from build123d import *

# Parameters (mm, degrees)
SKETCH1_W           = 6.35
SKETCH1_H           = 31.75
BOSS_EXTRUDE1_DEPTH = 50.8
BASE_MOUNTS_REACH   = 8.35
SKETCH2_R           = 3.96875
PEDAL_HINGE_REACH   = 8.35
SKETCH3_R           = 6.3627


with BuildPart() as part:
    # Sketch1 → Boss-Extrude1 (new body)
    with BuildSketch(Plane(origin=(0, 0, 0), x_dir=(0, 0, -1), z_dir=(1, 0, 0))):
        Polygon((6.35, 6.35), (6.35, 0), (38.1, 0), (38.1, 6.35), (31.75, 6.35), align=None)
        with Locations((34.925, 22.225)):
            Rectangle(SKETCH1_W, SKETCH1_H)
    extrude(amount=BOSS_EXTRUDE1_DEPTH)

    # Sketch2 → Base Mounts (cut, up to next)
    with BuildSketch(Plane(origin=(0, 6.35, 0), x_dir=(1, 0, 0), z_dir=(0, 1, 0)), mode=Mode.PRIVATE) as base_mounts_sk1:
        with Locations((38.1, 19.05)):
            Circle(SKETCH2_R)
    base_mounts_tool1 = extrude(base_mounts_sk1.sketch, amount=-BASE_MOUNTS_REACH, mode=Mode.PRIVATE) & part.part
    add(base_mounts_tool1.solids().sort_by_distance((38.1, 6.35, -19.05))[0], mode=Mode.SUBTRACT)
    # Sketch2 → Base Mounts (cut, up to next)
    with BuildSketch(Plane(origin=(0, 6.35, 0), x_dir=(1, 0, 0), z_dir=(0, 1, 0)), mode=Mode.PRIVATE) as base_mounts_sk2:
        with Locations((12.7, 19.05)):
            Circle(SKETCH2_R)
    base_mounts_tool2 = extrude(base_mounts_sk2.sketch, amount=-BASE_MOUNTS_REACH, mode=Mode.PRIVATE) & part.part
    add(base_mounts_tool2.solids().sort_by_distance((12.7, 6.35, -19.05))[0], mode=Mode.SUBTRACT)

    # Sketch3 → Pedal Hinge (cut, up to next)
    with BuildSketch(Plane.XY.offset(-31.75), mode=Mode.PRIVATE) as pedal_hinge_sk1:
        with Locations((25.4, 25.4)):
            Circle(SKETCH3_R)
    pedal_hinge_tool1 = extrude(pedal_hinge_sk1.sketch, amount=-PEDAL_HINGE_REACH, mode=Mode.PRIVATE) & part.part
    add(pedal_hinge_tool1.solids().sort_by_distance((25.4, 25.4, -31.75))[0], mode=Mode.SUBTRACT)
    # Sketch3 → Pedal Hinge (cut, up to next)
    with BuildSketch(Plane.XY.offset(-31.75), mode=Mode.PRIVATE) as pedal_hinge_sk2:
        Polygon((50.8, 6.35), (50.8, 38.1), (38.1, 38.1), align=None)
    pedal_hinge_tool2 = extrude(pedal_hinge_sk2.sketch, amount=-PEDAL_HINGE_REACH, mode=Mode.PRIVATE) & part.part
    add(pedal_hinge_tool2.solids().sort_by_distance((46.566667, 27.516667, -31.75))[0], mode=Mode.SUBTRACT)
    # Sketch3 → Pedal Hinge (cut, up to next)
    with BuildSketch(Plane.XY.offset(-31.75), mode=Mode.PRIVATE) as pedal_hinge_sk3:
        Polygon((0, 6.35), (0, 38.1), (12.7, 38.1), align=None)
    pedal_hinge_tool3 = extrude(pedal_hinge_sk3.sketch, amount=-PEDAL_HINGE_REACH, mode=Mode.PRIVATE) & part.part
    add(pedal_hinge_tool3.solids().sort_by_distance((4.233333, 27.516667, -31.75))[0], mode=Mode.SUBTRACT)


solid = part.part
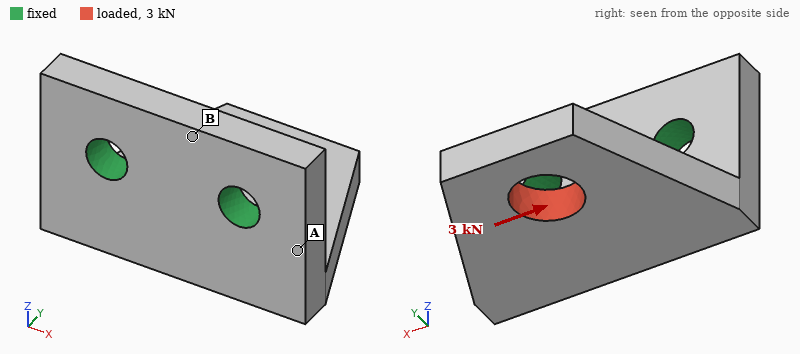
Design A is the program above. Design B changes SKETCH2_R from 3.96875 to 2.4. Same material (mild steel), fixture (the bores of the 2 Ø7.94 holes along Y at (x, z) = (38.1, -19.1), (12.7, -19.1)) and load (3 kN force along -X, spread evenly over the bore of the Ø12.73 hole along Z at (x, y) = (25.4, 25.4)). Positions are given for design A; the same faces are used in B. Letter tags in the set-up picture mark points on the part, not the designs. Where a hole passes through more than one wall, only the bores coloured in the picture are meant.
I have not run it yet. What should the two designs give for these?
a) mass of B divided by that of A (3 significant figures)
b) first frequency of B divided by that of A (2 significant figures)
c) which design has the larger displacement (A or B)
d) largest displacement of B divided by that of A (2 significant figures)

1.02
0.93
B
1.3
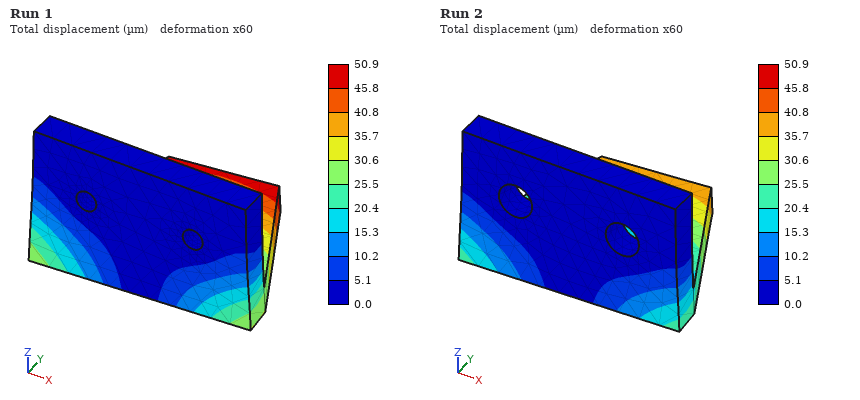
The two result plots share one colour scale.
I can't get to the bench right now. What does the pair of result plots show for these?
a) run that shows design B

Run 1
